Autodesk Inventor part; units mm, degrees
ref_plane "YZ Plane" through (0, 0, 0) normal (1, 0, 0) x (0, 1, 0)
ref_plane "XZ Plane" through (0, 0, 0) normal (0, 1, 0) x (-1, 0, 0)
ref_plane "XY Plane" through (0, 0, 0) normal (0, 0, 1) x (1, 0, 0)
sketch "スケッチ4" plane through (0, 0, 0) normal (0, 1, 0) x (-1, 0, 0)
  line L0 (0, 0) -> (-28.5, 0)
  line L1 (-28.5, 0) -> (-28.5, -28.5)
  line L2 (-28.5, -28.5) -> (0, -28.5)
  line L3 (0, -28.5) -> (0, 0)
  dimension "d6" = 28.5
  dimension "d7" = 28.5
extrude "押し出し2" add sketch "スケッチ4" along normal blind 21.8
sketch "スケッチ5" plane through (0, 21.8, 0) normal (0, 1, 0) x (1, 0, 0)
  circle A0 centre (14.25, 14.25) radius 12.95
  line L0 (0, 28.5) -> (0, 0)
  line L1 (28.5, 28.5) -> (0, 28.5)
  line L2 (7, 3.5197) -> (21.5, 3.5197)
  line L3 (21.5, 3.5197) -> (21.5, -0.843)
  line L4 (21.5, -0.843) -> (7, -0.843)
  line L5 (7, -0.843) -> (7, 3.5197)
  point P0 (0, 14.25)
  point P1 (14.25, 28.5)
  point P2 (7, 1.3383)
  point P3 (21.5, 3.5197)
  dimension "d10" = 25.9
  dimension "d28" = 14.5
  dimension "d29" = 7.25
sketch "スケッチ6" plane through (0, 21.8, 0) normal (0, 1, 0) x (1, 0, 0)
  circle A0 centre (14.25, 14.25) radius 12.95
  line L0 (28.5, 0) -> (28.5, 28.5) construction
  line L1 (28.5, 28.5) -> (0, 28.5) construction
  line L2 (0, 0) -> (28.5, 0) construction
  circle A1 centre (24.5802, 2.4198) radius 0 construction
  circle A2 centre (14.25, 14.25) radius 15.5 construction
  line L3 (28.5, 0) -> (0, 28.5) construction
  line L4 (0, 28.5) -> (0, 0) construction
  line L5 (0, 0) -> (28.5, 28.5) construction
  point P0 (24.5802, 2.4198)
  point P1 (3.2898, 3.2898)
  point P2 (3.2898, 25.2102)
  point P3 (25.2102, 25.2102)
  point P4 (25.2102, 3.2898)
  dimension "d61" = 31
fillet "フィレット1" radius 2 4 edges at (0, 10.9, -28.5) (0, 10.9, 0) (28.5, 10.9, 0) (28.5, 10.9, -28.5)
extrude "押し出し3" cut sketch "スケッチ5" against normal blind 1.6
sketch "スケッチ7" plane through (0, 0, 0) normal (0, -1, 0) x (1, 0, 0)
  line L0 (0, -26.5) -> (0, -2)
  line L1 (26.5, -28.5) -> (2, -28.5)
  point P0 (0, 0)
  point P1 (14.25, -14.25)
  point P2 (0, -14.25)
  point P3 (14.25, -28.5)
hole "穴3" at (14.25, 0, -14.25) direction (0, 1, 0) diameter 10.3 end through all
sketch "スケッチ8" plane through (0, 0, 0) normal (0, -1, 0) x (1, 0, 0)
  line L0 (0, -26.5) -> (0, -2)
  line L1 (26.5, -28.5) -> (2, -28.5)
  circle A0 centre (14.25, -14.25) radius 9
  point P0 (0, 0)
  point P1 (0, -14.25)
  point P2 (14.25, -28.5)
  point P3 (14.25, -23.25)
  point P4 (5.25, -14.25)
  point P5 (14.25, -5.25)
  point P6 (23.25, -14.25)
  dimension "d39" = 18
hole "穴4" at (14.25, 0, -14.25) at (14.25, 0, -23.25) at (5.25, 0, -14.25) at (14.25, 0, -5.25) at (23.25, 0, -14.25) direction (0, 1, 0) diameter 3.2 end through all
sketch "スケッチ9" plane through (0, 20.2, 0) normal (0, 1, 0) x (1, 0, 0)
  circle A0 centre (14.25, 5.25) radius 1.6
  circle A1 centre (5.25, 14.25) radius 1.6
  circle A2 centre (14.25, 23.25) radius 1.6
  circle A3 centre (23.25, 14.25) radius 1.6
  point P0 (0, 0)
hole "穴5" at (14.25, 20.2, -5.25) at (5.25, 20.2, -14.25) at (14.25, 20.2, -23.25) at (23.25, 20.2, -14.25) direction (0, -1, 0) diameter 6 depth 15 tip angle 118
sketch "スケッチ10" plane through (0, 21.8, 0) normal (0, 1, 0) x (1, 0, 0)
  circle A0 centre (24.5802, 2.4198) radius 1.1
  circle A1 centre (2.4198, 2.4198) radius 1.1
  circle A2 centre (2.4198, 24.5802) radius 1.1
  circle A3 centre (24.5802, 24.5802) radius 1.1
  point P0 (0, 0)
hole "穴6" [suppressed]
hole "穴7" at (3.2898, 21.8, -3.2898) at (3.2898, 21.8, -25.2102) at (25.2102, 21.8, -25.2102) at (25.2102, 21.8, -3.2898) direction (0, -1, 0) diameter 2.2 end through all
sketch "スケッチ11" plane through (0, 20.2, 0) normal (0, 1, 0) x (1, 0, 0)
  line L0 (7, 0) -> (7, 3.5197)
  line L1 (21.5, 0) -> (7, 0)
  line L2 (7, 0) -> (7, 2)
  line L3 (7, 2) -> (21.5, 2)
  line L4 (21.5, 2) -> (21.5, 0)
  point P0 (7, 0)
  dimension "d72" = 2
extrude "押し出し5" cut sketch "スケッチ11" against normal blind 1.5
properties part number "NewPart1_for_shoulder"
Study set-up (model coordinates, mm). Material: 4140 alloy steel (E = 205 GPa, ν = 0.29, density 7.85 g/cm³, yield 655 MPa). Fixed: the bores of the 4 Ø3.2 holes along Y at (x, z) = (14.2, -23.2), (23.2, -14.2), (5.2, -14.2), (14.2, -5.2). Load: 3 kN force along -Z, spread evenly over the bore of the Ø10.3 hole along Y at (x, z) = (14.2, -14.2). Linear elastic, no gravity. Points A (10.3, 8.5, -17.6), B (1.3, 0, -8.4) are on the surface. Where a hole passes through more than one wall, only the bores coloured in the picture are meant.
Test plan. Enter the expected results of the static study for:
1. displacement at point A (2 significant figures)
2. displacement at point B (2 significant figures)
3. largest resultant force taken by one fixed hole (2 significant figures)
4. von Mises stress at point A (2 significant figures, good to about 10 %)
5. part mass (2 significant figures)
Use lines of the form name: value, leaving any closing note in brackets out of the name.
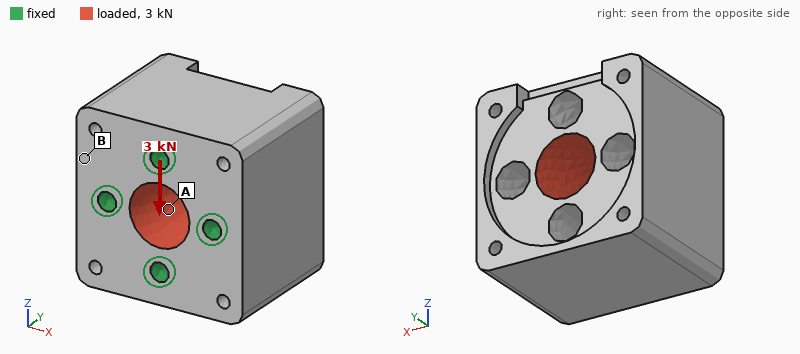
displacement at point A: 1.4 µm
displacement at point B: 0.60 µm
largest resultant force taken by one fixed hole: 1.2 kN
von Mises stress at point A: 21 MPa
part mass: 100 g
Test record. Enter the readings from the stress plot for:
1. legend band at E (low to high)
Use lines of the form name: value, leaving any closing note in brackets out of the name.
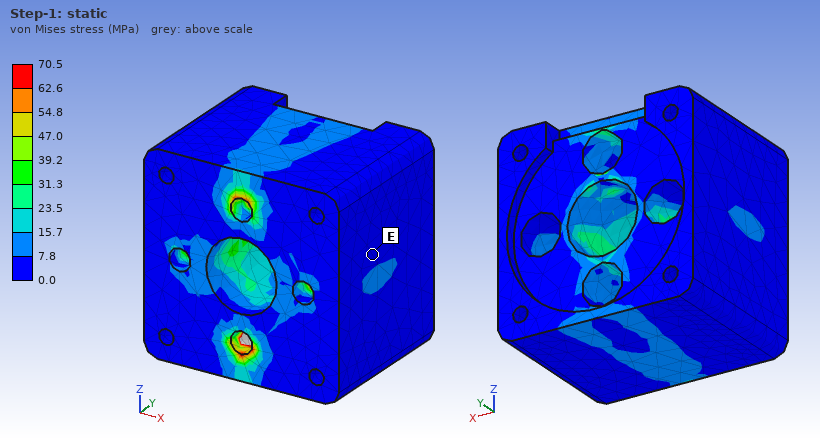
legend band at E: 0.0 to 7.8 MPa
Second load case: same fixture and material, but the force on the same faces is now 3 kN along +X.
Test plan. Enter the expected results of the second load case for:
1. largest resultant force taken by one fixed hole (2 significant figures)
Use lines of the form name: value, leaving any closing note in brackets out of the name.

largest resultant force taken by one fixed hole: 1.2 kN
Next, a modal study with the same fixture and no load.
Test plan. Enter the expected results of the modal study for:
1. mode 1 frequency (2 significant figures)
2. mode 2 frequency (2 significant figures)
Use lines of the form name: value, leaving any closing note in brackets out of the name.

mode 1 frequency: 16 kHz
mode 2 frequency: 16 kHz
